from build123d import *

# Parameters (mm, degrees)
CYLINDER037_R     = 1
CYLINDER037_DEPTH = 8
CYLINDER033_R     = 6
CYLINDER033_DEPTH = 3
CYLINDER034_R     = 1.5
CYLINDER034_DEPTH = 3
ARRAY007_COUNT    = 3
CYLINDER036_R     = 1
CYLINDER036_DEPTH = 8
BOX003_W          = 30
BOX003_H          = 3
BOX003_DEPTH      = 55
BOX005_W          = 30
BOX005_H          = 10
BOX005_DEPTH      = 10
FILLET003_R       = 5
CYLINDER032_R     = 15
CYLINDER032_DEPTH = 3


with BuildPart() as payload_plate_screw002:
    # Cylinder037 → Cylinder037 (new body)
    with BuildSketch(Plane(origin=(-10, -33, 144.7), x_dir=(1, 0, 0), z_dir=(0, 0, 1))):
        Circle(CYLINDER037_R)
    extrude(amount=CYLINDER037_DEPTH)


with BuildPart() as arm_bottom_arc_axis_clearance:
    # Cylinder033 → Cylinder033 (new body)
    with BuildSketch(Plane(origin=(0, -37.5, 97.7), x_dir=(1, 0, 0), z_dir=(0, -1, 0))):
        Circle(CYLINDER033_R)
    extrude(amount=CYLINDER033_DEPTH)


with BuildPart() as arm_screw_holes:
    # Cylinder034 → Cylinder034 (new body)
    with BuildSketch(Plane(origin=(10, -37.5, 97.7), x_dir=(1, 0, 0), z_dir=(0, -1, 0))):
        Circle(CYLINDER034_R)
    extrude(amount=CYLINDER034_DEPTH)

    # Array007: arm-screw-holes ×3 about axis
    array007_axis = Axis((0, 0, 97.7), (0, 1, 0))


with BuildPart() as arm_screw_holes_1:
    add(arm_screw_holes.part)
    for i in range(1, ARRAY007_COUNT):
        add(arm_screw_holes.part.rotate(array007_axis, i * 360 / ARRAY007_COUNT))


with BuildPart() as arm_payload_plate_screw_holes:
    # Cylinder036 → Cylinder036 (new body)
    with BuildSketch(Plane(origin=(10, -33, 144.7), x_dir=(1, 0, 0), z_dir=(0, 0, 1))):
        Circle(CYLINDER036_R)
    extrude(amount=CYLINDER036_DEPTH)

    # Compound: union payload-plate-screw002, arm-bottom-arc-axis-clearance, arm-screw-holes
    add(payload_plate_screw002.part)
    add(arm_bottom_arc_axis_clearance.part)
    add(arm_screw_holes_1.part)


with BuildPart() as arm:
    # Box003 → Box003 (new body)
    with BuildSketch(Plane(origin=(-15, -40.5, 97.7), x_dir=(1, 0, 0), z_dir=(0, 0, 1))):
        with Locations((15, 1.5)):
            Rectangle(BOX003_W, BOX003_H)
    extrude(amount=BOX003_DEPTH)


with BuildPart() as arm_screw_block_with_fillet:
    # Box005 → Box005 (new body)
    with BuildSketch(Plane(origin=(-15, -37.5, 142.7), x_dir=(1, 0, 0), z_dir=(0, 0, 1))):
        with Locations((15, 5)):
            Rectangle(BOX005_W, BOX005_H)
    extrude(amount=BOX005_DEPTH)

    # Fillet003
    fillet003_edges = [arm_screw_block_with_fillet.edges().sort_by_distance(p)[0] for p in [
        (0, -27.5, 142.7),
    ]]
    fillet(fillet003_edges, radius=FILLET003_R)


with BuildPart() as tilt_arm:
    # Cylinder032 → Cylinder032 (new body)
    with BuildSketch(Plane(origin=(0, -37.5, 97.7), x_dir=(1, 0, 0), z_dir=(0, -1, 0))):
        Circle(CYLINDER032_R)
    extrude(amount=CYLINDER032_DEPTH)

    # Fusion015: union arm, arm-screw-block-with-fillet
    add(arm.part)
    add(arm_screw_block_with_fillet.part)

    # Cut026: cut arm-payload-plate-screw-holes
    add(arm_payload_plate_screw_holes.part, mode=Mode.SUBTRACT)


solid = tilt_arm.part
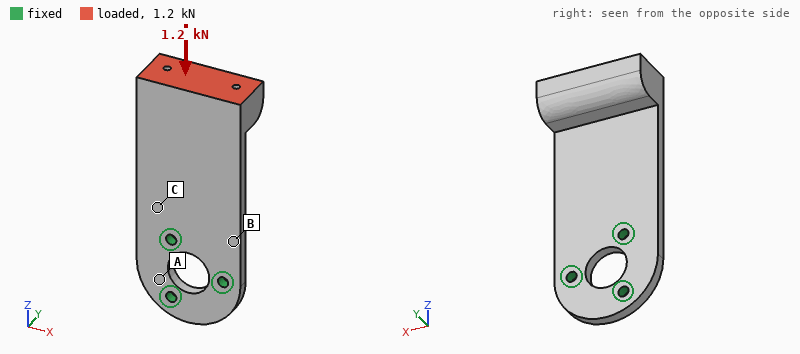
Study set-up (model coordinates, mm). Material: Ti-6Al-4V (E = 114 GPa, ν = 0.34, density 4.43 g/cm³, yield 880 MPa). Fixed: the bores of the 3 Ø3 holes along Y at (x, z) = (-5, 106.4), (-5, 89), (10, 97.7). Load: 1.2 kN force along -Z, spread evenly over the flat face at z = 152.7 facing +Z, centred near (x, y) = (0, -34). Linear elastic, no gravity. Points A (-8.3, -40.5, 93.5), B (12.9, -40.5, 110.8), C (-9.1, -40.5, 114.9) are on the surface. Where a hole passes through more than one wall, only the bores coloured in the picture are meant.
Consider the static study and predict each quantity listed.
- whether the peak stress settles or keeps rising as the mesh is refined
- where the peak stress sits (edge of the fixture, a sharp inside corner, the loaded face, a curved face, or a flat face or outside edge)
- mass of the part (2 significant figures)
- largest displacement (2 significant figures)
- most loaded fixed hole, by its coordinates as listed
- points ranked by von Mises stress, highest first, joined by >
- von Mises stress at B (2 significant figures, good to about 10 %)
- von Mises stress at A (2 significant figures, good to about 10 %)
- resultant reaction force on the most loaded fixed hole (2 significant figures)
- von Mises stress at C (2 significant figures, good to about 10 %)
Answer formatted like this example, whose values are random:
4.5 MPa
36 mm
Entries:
keeps rising
edge of the fixture
37 g
0.92 mm
(-5, 106.4)
C > B > A
90 MPa
23 MPa
690 N
120 MPa
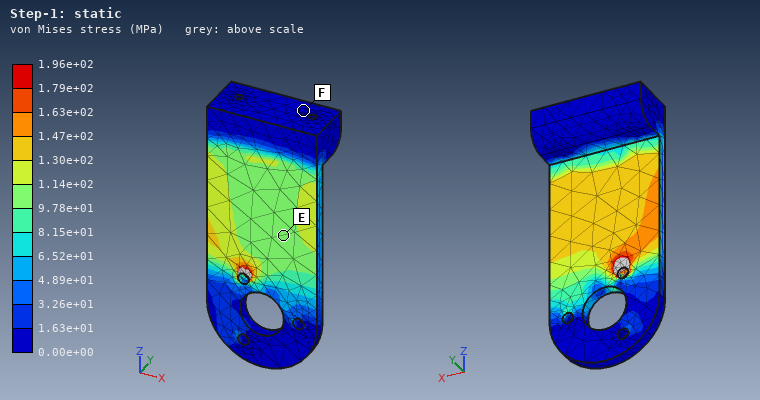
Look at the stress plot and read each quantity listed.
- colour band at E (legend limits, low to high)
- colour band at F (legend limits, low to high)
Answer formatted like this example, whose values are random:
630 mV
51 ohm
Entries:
9.78e+01 to 1.14e+02 MPa
0.00e+00 to 1.63e+01 MPa
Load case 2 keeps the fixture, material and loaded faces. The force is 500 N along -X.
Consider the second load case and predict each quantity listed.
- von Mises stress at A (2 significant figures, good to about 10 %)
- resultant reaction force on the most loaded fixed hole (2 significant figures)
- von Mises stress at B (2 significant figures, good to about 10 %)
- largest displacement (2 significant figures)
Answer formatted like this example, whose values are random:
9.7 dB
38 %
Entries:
22 MPa
1.2 kN
66 MPa
0.18 mm
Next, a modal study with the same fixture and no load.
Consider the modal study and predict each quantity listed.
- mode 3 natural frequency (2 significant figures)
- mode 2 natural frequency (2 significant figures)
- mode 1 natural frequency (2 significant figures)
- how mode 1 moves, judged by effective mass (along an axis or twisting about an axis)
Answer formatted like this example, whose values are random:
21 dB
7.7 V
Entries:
4300 Hz
2000 Hz
620 Hz
along Y
